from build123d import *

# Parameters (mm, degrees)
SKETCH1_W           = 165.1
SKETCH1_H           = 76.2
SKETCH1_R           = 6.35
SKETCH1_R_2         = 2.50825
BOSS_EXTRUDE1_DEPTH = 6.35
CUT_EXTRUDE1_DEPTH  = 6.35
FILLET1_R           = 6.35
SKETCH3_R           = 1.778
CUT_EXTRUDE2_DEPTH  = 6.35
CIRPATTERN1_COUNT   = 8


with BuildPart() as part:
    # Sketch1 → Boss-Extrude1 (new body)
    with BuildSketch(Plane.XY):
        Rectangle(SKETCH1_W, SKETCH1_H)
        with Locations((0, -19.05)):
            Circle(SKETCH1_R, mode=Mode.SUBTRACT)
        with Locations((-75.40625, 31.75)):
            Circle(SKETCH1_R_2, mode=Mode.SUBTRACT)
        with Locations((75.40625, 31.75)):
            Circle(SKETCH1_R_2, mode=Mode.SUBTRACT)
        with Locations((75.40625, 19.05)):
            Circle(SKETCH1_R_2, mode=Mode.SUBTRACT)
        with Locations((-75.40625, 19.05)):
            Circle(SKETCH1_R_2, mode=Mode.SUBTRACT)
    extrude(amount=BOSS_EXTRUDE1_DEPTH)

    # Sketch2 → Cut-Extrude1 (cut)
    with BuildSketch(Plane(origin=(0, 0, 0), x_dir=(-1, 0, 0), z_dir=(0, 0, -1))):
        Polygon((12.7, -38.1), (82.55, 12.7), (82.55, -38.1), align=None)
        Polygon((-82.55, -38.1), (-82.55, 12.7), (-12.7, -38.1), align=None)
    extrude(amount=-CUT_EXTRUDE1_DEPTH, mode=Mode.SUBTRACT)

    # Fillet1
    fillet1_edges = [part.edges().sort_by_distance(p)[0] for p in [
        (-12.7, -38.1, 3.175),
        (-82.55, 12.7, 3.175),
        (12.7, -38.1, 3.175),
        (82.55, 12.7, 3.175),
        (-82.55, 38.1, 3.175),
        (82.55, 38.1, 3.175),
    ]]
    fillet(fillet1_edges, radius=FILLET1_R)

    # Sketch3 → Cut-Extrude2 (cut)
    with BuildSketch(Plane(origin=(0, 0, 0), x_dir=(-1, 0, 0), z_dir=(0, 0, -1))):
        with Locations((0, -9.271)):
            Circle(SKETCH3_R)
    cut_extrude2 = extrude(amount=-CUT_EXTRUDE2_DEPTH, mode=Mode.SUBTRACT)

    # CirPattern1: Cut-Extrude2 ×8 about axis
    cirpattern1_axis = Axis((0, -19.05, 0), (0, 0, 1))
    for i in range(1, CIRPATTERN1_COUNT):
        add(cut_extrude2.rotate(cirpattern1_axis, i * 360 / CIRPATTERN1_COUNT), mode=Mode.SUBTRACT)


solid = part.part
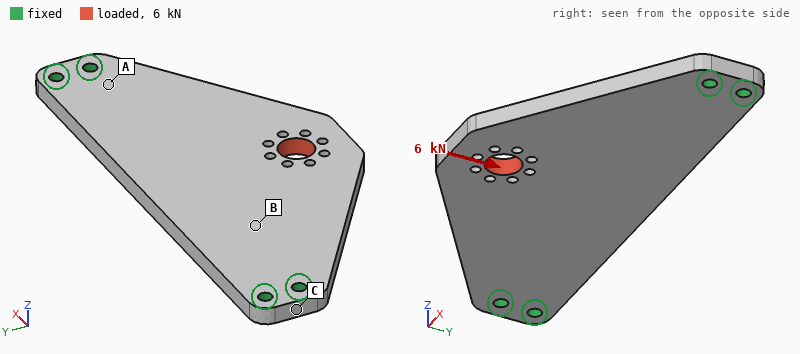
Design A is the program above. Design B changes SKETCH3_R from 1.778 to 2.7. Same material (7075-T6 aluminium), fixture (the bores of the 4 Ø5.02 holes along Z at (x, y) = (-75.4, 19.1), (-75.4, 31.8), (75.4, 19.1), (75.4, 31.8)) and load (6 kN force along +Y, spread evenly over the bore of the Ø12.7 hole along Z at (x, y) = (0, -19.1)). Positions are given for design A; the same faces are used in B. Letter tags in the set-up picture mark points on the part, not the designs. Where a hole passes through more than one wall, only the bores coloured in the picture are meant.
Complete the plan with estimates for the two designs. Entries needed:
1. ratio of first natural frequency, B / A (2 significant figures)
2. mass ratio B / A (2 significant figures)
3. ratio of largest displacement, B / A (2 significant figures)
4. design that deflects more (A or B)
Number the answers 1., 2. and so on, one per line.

1. 1.0
2. 0.99
3. 1.2
4. B
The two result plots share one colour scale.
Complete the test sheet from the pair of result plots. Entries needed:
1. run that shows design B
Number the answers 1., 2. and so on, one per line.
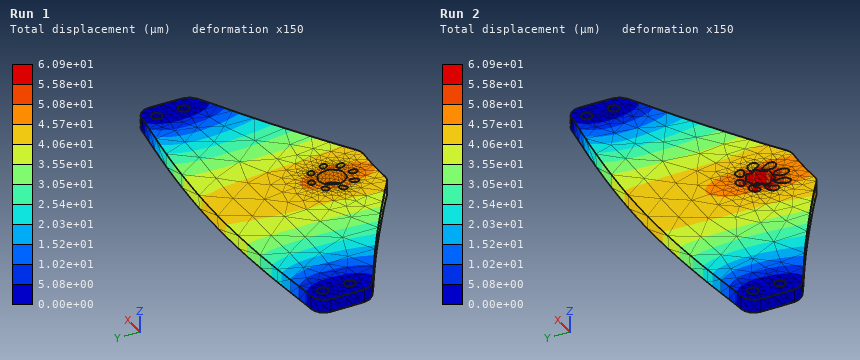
1. Run 2
